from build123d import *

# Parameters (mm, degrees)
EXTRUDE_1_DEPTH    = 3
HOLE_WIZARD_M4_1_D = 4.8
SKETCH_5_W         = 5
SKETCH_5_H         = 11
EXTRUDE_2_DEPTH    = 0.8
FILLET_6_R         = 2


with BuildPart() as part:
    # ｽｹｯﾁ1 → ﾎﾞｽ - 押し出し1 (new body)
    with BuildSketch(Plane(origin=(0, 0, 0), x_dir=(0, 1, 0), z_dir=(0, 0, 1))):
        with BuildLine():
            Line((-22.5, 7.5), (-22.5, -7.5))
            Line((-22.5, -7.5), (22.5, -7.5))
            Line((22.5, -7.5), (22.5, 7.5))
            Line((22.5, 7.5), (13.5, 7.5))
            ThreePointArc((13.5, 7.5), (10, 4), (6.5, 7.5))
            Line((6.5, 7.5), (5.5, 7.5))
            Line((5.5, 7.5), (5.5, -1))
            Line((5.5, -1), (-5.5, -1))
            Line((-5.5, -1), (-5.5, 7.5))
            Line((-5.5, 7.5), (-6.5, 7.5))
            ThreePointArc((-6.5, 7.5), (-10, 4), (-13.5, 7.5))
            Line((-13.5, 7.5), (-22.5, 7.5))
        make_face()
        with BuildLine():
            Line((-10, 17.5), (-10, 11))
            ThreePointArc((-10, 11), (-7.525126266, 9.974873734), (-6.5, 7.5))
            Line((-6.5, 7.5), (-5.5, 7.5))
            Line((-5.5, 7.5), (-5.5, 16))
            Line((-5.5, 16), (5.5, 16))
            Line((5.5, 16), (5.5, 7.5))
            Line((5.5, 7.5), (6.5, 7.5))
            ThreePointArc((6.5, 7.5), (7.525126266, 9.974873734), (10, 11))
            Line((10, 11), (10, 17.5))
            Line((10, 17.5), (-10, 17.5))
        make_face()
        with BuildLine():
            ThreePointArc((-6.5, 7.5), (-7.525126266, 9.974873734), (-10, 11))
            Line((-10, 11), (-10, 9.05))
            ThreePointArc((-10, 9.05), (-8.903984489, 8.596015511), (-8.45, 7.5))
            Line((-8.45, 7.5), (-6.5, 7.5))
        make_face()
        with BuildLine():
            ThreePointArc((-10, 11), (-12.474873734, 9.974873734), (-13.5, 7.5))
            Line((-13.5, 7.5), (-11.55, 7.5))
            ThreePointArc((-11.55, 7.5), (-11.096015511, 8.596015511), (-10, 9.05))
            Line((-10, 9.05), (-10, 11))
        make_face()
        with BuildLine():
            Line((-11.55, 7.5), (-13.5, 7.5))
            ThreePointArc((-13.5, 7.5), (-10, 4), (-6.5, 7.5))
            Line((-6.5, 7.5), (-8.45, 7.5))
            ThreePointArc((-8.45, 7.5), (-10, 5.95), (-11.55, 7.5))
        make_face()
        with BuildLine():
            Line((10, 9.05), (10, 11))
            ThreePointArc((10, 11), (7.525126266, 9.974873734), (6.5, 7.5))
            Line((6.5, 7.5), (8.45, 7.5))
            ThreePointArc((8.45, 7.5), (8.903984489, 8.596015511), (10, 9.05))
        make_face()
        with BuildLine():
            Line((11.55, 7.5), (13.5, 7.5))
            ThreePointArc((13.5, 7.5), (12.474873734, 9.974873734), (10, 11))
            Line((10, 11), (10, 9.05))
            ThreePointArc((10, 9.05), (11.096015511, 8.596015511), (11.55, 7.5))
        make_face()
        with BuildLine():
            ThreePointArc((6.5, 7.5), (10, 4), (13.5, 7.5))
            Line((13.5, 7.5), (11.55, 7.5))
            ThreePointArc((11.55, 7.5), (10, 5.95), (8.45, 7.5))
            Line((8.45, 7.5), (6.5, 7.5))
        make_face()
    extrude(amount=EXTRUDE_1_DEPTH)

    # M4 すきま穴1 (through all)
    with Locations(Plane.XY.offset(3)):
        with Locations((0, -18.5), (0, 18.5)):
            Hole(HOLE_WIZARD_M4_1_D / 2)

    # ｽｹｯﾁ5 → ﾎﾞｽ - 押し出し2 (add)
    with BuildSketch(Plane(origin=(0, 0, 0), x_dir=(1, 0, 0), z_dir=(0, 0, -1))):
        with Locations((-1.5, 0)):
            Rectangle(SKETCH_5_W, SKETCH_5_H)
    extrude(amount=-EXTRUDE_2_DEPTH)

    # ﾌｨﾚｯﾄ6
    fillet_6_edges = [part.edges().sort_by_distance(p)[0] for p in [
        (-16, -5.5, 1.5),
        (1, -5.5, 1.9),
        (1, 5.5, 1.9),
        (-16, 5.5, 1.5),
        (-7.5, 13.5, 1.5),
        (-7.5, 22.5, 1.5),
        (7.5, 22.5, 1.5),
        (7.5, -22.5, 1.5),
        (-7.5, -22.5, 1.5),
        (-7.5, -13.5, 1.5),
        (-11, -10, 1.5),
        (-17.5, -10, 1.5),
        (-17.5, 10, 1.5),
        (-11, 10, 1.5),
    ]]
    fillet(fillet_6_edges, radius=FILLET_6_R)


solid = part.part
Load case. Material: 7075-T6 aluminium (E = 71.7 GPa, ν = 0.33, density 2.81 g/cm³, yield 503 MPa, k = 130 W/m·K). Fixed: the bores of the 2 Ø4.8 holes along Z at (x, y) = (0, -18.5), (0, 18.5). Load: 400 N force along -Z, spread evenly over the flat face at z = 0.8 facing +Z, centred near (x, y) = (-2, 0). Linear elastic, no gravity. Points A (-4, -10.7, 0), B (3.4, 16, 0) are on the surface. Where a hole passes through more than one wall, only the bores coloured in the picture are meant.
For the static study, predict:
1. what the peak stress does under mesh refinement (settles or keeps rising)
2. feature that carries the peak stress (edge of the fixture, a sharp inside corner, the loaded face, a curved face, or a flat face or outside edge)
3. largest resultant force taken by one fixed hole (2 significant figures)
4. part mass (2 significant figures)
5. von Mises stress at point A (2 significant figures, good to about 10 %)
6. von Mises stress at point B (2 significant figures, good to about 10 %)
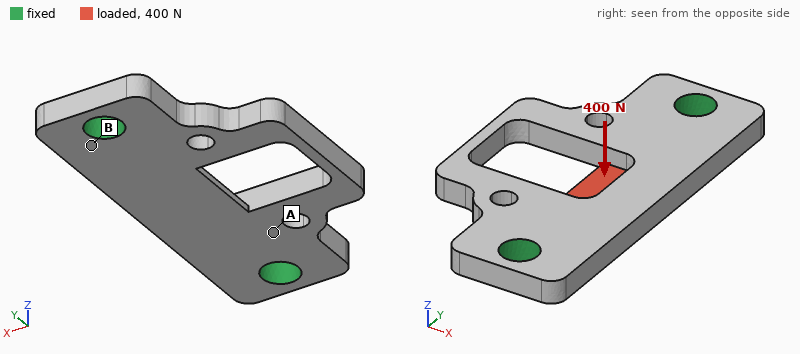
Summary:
keeps rising
a sharp inside corner
250 N
5.7 g
23 MPa
43 MPa
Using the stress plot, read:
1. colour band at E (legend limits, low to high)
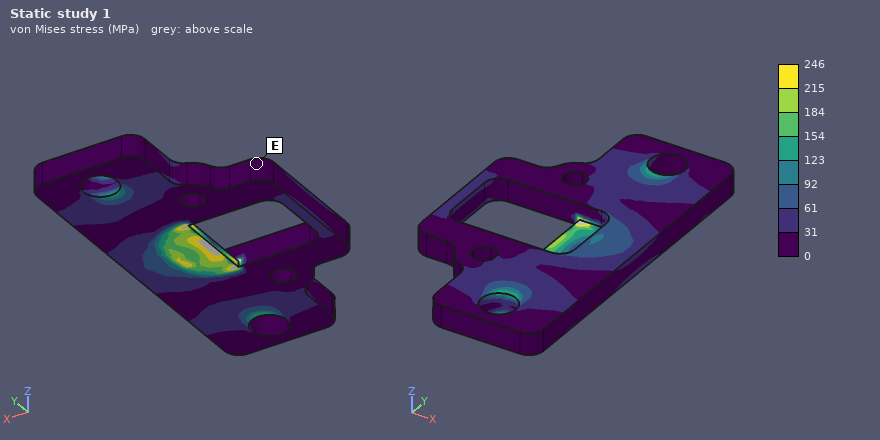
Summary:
0 to 31 MPa
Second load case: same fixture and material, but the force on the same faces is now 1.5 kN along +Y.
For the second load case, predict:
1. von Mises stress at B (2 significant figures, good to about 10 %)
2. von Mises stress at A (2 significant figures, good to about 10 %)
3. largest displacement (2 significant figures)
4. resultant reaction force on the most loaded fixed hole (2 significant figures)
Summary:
21 MPa
39 MPa
18 µm
760 N
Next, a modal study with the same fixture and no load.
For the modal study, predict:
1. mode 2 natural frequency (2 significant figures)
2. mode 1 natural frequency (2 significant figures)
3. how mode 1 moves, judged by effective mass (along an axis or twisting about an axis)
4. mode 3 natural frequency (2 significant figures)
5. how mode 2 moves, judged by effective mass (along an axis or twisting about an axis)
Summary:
13 kHz
7600 Hz
along Z
15 kHz
along Z
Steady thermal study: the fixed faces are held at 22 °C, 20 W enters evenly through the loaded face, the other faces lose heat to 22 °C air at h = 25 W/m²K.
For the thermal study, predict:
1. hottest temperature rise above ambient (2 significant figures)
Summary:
61 K
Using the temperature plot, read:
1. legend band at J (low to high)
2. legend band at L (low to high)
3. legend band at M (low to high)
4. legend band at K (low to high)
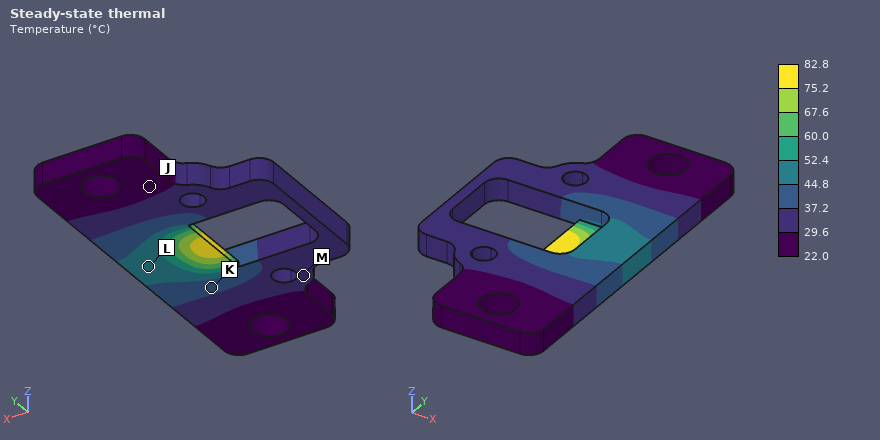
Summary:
22.0 to 29.6 °C
44.8 to 52.4 °C
29.6 to 37.2 °C
37.2 to 44.8 °C
